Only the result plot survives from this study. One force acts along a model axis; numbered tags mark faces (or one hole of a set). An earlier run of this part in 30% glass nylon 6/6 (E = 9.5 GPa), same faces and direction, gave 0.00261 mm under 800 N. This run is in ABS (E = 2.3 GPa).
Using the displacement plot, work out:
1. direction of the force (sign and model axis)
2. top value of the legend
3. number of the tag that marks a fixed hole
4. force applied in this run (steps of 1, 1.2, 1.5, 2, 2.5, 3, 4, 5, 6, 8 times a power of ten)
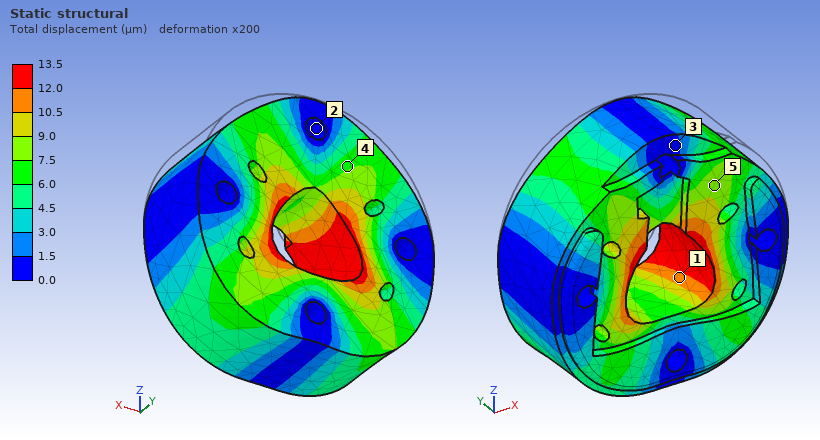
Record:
-Z
13.5 µm
2
1 kN
